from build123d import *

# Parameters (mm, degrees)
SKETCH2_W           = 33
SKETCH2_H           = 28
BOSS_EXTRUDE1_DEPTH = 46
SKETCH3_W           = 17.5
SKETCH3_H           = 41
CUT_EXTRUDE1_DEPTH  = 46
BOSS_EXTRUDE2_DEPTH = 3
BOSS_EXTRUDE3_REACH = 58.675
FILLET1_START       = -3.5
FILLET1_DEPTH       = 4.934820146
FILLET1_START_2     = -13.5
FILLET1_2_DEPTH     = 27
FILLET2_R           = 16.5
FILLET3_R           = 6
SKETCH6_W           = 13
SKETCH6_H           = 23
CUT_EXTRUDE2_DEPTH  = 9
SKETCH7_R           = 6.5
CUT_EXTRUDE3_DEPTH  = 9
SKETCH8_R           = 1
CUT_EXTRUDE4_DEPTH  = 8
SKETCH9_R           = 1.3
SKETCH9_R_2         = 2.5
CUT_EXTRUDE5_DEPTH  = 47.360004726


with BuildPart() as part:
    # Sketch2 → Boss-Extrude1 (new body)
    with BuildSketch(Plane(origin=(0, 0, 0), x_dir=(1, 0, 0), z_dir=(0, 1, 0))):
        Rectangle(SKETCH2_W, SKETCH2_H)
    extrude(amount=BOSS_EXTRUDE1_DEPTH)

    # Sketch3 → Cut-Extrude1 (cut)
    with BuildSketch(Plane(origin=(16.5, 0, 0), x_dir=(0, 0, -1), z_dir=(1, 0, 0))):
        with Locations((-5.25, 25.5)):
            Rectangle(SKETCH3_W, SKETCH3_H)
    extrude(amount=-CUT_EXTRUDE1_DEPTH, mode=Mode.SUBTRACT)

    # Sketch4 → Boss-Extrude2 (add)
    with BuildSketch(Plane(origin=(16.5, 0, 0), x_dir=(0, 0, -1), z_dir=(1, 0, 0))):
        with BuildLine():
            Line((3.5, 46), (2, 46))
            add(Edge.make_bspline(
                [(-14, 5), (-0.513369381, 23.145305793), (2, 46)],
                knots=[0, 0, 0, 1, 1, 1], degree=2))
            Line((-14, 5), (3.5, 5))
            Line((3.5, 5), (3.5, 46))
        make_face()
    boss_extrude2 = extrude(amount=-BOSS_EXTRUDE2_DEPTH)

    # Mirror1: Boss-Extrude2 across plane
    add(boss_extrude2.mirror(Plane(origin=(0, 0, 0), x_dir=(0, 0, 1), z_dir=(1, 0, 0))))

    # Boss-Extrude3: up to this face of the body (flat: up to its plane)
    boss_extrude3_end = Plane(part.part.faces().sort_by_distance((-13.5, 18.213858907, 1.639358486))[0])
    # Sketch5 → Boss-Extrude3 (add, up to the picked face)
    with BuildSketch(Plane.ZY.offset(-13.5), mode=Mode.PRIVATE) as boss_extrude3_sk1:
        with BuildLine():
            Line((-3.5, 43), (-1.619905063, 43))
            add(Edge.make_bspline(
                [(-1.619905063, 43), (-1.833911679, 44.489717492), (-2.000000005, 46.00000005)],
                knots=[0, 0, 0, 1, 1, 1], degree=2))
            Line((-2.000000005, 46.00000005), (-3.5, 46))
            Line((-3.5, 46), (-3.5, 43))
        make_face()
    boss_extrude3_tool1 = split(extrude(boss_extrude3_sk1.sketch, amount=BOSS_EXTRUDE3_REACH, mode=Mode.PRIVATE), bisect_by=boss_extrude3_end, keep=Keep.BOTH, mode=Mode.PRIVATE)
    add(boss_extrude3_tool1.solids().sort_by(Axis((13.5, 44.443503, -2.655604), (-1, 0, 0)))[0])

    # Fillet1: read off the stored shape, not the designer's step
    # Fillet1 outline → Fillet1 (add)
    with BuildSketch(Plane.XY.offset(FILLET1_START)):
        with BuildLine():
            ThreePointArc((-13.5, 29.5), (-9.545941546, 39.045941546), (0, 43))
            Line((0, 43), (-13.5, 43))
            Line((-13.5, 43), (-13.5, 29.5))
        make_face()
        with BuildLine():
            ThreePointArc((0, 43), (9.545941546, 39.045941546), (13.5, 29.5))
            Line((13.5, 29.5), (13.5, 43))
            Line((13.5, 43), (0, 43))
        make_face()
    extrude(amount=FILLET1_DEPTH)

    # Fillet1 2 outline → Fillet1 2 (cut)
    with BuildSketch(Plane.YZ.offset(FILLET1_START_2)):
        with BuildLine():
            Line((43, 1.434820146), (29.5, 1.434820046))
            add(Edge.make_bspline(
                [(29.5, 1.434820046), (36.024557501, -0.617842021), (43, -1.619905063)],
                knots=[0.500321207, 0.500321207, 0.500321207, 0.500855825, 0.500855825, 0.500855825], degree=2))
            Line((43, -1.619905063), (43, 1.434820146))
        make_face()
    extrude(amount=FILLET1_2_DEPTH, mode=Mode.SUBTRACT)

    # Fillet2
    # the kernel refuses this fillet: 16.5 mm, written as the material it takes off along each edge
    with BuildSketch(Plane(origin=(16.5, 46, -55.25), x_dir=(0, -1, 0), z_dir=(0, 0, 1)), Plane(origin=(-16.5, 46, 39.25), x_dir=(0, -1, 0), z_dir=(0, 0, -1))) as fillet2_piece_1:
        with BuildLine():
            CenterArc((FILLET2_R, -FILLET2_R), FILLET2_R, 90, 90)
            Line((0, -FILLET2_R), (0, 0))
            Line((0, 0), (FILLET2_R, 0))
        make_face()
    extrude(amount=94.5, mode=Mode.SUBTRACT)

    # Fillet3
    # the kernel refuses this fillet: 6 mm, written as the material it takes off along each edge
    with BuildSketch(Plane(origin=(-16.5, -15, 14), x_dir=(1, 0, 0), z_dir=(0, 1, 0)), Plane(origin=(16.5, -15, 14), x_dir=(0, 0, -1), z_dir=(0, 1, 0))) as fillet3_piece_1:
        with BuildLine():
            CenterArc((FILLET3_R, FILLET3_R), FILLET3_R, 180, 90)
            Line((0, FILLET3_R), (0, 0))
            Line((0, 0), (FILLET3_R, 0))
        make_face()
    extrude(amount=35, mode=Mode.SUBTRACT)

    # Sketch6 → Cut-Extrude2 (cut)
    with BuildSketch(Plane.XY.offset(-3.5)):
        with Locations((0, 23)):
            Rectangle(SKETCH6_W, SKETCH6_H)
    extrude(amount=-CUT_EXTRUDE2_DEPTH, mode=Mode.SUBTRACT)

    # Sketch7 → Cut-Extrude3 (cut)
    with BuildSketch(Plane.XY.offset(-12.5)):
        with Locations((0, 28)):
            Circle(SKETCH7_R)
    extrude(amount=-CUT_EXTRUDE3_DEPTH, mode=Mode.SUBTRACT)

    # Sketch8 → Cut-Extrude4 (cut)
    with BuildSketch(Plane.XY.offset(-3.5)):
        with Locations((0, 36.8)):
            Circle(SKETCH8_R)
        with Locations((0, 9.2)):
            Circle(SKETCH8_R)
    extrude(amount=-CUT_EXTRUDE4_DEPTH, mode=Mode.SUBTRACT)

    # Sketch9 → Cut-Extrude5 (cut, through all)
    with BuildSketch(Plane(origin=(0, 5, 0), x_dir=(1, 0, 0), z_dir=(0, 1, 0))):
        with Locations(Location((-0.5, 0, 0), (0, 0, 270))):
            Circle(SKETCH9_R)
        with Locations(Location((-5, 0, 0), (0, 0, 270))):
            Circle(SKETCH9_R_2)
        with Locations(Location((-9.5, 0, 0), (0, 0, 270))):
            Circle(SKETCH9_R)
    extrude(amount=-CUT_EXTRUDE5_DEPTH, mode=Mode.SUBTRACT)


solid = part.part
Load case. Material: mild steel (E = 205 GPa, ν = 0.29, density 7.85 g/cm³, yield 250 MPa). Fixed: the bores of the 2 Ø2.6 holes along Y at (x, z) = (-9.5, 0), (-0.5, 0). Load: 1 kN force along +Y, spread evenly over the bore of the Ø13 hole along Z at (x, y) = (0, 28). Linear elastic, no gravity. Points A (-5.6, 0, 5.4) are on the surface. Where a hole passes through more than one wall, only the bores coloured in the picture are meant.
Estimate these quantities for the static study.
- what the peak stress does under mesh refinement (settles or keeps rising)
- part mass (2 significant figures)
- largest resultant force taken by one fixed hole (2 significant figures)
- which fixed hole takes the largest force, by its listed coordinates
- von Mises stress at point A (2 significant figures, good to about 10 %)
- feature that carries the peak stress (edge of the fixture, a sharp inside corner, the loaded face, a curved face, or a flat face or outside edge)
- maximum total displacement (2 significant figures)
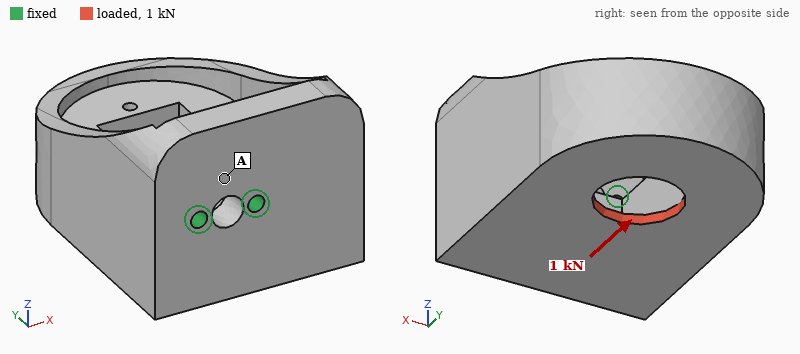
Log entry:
keeps rising
130 g
820 N
(-0.5, 0)
19 MPa
edge of the fixture
41 µm
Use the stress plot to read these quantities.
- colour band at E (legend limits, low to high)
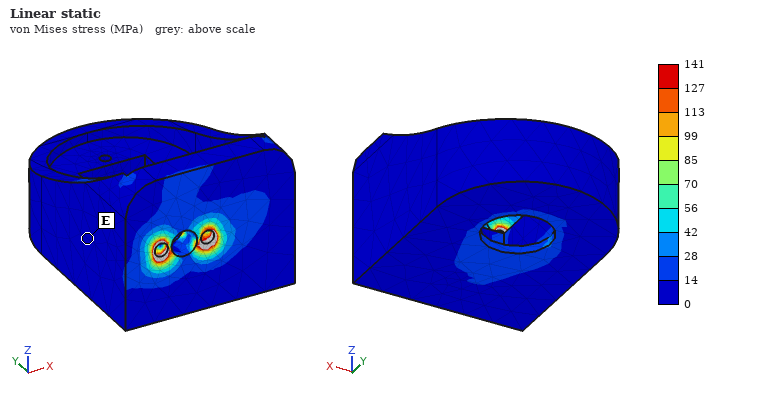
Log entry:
0 to 14 MPa
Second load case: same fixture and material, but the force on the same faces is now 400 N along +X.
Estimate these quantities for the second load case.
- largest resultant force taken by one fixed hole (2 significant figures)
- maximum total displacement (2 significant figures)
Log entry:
860 N
15 µm
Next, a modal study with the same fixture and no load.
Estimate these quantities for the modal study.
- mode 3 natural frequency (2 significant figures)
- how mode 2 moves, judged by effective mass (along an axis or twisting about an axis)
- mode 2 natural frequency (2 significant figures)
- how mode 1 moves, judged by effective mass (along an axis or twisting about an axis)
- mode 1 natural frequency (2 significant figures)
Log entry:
7600 Hz
along X
3300 Hz
along Z
2400 Hz
